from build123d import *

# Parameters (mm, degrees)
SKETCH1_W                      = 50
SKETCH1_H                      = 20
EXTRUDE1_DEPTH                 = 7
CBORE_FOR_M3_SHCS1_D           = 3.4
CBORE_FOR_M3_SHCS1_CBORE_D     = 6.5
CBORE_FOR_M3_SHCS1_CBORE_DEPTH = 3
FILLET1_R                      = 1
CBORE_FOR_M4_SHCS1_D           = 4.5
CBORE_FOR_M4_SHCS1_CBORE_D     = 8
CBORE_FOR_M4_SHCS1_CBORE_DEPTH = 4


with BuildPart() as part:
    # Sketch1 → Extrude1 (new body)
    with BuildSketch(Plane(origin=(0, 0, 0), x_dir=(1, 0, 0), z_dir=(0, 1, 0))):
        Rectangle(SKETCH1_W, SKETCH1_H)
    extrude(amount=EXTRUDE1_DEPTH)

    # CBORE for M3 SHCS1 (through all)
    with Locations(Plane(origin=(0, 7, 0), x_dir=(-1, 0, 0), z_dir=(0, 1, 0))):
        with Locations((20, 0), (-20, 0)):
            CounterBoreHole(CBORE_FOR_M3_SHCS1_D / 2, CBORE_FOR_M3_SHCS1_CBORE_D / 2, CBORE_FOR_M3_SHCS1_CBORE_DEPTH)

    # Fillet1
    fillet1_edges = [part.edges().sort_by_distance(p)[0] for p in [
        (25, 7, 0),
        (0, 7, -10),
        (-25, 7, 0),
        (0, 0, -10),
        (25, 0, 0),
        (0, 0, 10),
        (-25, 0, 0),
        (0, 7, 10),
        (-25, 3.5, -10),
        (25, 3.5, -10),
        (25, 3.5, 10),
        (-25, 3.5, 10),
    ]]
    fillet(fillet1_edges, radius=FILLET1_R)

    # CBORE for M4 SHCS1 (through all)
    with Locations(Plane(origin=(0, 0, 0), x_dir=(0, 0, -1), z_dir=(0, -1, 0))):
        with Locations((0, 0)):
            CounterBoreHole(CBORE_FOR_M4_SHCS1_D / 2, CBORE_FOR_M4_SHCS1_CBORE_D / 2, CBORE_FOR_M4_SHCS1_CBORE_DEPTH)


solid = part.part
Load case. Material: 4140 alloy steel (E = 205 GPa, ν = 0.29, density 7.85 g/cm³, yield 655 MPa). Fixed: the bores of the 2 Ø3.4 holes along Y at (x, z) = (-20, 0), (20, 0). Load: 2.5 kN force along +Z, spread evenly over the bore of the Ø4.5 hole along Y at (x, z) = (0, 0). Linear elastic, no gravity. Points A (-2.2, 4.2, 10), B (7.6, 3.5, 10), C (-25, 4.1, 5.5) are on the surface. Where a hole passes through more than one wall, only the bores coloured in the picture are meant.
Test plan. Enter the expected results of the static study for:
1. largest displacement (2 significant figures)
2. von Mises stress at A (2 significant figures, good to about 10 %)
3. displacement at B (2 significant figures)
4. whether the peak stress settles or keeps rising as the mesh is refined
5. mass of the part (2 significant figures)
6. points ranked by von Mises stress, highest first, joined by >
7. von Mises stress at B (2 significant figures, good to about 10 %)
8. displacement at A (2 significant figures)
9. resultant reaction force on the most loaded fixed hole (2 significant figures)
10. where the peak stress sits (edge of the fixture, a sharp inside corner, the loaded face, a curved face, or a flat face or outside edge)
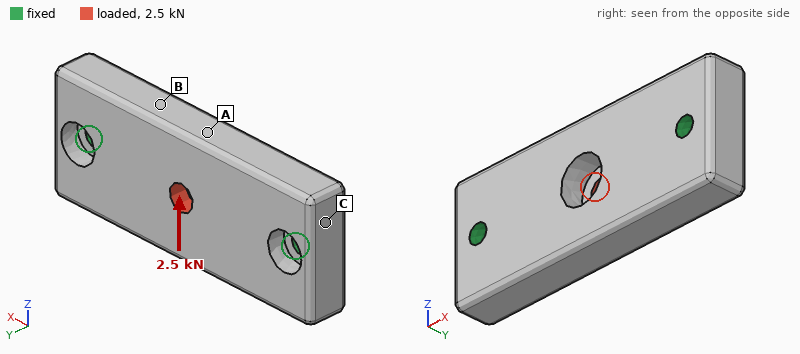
11 µm
49 MPa
8.4 µm
keeps rising
50 g
A > B > C
33 MPa
9.7 µm
1.3 kN
edge of the fixture
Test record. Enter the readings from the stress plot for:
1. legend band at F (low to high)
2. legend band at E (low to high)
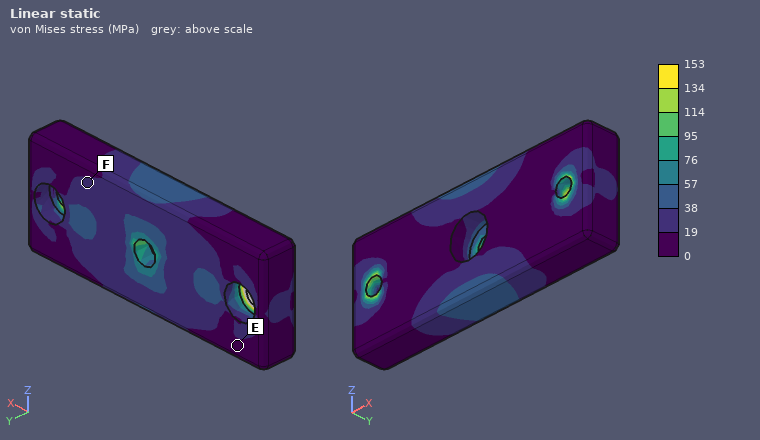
19 to 38 MPa
0 to 19 MPa
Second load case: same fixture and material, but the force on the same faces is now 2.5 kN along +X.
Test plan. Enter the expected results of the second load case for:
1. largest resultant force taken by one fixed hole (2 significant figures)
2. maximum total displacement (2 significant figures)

1.3 kN
2.6 µm
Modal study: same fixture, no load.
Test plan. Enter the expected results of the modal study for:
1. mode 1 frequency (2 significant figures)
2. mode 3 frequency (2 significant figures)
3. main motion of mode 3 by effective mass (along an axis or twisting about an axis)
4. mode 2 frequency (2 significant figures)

14 kHz
24 kHz
along Z
14 kHz
